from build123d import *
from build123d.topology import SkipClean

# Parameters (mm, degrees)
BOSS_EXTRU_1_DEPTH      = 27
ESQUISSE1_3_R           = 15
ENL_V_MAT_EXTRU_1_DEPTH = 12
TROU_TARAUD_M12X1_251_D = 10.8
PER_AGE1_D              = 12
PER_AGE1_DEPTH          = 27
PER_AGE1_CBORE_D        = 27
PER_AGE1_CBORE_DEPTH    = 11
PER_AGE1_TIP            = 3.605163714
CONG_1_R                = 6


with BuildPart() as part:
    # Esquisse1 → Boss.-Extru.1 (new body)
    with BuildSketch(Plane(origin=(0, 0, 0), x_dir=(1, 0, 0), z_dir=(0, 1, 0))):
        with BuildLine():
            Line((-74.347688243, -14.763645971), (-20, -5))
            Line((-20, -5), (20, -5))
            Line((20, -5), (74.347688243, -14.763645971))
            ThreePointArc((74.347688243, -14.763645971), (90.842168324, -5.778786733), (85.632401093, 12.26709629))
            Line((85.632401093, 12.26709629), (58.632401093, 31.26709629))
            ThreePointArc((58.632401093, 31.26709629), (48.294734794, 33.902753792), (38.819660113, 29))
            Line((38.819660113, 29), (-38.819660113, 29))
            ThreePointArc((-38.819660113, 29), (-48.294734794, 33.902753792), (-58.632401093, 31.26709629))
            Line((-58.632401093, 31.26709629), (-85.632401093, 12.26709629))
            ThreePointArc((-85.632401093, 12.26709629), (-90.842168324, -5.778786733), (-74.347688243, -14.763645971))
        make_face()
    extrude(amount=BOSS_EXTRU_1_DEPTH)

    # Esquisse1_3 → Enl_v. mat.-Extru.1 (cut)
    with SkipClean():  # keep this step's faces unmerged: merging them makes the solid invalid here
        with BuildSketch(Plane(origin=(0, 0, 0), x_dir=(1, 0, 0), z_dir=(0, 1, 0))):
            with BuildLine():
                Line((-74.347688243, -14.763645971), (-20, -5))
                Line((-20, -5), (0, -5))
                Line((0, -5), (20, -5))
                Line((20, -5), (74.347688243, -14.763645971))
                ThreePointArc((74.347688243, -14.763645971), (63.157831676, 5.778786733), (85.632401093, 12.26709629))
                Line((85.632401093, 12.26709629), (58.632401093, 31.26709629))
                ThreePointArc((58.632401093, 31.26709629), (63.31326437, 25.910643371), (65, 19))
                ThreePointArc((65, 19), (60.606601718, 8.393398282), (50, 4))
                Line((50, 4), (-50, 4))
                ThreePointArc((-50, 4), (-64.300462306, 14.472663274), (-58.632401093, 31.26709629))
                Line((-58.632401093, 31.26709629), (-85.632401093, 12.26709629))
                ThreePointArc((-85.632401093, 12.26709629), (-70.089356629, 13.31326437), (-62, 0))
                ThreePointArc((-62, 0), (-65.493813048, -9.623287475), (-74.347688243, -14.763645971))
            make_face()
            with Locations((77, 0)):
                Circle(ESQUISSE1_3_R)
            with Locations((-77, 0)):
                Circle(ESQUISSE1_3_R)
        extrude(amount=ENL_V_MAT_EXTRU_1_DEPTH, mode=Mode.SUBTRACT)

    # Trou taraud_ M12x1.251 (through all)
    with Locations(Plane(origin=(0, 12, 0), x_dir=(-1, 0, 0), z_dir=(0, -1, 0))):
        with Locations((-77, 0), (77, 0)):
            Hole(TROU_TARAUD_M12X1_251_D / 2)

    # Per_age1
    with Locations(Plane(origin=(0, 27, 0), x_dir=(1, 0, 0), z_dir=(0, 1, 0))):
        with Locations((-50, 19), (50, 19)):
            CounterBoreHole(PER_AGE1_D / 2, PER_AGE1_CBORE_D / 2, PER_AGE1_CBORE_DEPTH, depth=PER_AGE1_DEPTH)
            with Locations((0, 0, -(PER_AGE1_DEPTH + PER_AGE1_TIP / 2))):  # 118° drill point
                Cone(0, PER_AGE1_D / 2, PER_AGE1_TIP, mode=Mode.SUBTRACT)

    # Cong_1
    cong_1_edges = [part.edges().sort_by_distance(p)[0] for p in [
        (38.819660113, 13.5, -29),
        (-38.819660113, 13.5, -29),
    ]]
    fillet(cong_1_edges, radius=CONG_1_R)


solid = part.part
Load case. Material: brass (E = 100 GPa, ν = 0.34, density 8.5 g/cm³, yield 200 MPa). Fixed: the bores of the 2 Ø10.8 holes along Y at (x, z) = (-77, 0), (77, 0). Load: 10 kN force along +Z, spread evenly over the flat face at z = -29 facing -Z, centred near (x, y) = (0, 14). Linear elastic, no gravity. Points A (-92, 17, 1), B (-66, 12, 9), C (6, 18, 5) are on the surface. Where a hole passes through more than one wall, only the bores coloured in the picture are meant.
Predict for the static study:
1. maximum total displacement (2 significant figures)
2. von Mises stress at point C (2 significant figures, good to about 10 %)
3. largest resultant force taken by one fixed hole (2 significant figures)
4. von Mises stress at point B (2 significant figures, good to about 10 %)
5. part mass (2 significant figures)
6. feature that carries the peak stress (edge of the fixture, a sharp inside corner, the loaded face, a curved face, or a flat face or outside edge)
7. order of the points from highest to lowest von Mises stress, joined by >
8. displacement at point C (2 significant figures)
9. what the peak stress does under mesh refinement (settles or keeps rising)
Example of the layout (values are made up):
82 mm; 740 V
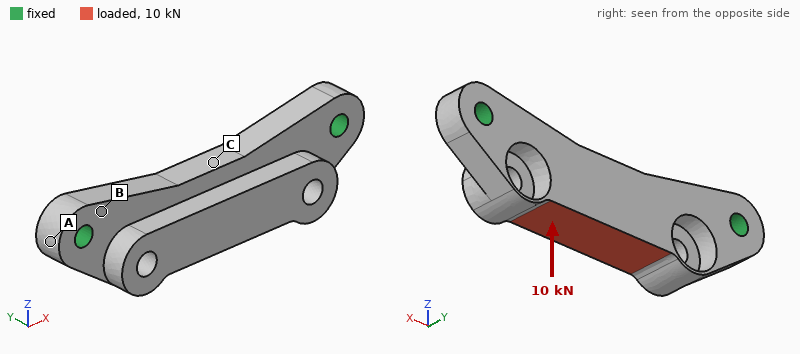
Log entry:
74 µm; 27 MPa; 6.8 kN; 40 MPa; 1.0 kg; edge of the fixture; B > C > A; 53 µm; keeps rising
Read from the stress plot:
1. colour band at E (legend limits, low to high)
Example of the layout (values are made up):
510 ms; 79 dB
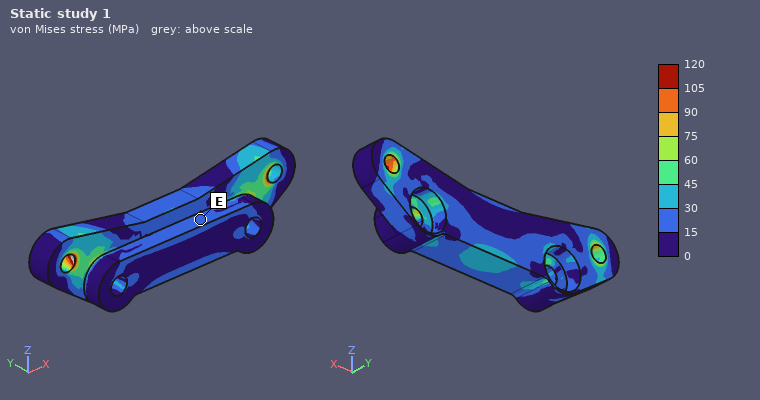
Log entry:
15 to 30 MPa
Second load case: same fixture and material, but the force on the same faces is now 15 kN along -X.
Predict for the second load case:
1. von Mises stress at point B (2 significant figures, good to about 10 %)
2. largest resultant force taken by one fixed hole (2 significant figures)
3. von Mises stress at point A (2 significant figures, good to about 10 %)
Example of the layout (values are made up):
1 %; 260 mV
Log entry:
21 MPa; 8.1 kN; 5.6 MPa
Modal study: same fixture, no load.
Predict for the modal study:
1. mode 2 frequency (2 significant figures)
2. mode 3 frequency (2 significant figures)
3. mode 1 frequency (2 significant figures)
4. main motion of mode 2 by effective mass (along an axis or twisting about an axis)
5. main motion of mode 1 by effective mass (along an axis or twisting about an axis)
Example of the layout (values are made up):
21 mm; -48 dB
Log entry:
3100 Hz; 3900 Hz; 2000 Hz; along Z; along Y
